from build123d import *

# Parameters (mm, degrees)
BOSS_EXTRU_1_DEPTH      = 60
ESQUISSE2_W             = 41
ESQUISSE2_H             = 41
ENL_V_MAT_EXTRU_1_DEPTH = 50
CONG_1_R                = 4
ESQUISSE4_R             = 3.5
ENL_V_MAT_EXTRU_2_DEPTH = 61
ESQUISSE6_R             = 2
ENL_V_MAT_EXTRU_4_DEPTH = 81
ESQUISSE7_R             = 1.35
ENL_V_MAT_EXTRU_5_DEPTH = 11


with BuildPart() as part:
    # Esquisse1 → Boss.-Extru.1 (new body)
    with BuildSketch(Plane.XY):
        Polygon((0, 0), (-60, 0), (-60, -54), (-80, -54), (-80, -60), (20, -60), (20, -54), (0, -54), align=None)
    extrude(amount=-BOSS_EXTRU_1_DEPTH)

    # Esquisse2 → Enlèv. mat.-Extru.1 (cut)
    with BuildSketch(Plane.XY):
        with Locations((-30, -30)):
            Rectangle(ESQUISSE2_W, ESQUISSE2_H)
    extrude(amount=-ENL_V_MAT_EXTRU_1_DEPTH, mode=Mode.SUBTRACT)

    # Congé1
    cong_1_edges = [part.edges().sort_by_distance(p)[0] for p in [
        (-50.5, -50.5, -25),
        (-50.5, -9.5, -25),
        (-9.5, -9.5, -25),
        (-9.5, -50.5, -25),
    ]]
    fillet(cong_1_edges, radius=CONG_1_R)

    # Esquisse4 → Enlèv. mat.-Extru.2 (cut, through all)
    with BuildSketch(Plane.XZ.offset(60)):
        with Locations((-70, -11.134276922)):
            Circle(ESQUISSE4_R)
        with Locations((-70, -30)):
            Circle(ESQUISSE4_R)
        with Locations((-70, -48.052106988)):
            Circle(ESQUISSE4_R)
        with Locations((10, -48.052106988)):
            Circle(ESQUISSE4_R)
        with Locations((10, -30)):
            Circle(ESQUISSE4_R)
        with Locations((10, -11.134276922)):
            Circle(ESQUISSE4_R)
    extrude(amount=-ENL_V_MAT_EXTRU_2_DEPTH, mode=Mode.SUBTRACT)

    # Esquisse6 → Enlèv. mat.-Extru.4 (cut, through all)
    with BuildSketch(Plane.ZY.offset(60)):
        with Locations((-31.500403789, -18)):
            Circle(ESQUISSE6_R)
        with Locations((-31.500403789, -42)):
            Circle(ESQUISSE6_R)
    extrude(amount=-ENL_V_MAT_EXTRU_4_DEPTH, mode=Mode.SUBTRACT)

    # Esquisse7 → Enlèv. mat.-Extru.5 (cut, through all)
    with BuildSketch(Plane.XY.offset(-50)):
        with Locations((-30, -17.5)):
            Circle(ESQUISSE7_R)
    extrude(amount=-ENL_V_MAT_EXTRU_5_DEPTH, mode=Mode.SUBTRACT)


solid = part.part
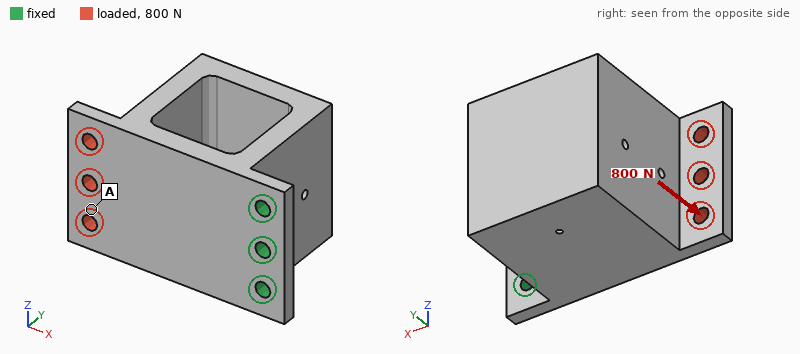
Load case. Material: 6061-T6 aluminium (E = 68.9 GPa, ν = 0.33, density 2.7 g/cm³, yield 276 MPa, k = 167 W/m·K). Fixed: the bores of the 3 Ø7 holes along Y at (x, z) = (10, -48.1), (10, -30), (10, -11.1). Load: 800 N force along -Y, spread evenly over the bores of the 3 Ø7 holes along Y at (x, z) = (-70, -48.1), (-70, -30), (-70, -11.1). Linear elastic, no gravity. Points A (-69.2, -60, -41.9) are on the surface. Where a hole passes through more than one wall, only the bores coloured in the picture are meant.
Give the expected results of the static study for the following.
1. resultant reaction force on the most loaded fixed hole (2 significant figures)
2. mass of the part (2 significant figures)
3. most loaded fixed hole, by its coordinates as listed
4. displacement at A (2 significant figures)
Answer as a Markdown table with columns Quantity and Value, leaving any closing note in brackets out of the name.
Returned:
| Quantity | Value |
|---|---|
| resultant reaction force on the most loaded fixed hole | 340 N |
| mass of the part | 390 g |
| most loaded fixed hole, by its coordinates as listed | (10, -30) |
| displacement at A | 0.66 mm |
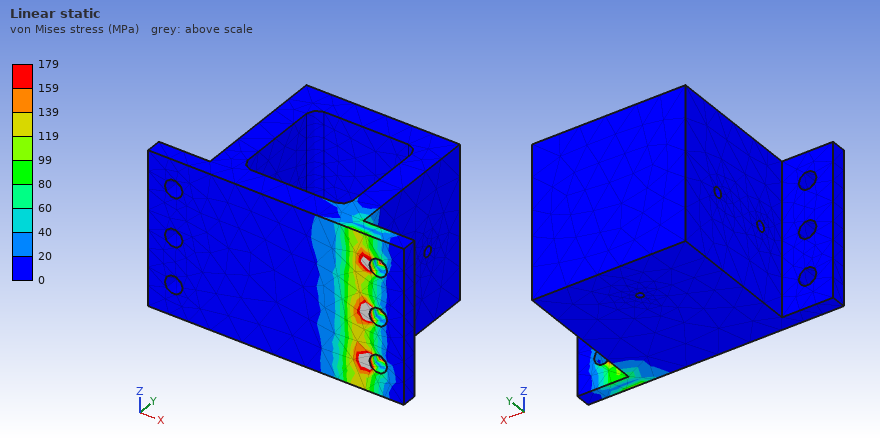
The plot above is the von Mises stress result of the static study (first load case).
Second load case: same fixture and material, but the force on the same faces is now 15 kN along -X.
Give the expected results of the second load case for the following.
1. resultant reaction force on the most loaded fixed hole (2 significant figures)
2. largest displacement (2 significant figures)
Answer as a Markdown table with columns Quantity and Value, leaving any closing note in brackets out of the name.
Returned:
| Quantity | Value |
|---|---|
| resultant reaction force on the most loaded fixed hole | 5.3 kN |
| largest displacement | 0.12 mm |
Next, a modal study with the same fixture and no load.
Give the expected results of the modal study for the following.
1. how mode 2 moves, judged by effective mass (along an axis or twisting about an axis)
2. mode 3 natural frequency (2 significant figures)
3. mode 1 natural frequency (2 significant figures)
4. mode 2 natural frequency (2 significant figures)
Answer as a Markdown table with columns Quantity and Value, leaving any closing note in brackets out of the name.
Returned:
| Quantity | Value |
|---|---|
| how mode 2 moves, judged by effective mass | along Z |
| mode 3 natural frequency | 3100 Hz |
| mode 1 natural frequency | 400 Hz |
| mode 2 natural frequency | 1700 Hz |
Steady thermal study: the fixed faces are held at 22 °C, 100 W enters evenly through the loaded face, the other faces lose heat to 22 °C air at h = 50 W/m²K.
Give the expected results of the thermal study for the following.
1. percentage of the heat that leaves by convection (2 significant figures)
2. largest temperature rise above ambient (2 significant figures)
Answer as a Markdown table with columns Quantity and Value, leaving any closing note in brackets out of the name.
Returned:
| Quantity | Value |
|---|---|
| percentage of the heat that leaves by convection | 41 % |
| largest temperature rise above ambient | 66 K |
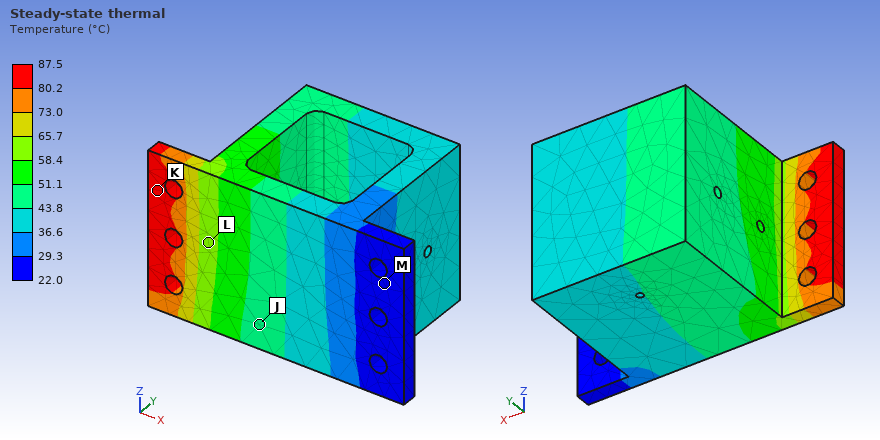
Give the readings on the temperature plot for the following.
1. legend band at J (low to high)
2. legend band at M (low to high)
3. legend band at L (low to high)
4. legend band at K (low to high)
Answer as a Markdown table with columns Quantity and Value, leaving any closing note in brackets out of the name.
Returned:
| Quantity | Value |
|---|---|
| legend band at J | 43.8 to 51.1 °C |
| legend band at M | 22.0 to 29.3 °C |
| legend band at L | 58.4 to 65.7 °C |
| legend band at K | 80.2 to 87.5 °C |
